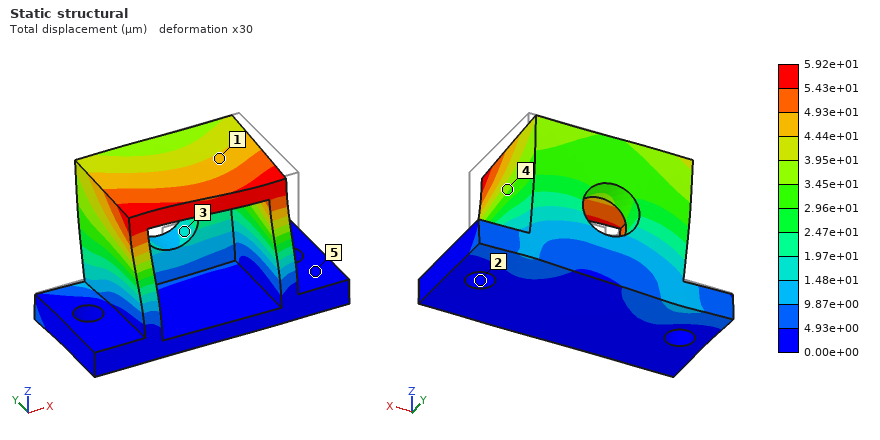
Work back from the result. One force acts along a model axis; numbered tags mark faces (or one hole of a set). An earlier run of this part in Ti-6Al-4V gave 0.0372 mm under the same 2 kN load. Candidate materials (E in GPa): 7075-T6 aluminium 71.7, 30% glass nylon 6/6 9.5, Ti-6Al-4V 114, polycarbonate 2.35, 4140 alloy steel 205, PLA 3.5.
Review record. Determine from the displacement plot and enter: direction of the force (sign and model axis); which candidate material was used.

-X
7075-T6 aluminium
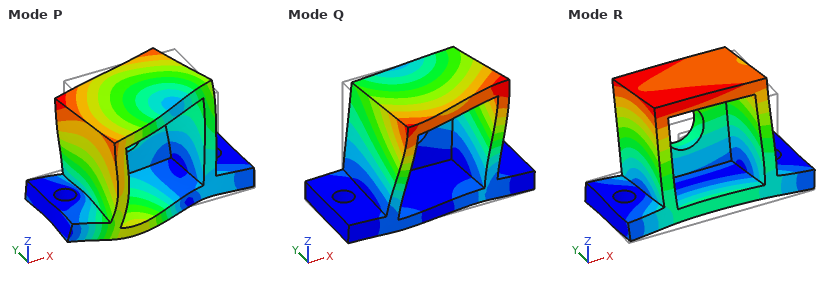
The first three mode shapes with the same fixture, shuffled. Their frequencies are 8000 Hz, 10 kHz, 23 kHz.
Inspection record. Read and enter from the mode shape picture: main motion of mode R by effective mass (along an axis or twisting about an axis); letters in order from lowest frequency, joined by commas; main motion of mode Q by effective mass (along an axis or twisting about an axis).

along Y
R, Q, P
along X
